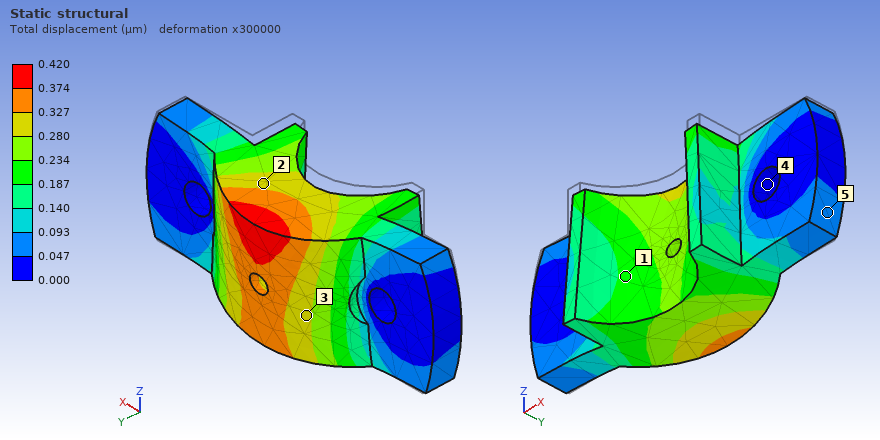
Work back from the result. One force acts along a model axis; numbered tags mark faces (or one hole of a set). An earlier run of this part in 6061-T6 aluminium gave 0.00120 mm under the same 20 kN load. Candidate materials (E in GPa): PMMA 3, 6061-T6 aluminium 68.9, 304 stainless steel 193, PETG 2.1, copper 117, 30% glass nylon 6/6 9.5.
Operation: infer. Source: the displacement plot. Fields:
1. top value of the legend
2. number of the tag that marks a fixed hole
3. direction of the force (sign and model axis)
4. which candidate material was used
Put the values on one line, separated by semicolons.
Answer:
0.420 µm; 4; -Z; 304 stainless steel
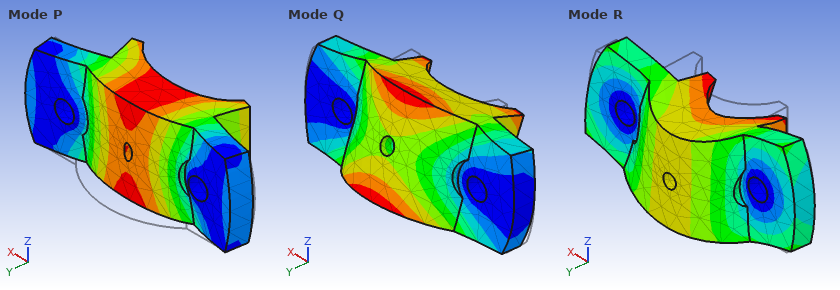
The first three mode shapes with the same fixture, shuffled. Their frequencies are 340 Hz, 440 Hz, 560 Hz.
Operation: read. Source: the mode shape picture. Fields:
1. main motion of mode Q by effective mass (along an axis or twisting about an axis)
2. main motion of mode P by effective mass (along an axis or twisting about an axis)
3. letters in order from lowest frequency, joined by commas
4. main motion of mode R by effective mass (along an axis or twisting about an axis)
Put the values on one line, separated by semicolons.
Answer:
twisting about X; along Y; Q, P, R; along Z
